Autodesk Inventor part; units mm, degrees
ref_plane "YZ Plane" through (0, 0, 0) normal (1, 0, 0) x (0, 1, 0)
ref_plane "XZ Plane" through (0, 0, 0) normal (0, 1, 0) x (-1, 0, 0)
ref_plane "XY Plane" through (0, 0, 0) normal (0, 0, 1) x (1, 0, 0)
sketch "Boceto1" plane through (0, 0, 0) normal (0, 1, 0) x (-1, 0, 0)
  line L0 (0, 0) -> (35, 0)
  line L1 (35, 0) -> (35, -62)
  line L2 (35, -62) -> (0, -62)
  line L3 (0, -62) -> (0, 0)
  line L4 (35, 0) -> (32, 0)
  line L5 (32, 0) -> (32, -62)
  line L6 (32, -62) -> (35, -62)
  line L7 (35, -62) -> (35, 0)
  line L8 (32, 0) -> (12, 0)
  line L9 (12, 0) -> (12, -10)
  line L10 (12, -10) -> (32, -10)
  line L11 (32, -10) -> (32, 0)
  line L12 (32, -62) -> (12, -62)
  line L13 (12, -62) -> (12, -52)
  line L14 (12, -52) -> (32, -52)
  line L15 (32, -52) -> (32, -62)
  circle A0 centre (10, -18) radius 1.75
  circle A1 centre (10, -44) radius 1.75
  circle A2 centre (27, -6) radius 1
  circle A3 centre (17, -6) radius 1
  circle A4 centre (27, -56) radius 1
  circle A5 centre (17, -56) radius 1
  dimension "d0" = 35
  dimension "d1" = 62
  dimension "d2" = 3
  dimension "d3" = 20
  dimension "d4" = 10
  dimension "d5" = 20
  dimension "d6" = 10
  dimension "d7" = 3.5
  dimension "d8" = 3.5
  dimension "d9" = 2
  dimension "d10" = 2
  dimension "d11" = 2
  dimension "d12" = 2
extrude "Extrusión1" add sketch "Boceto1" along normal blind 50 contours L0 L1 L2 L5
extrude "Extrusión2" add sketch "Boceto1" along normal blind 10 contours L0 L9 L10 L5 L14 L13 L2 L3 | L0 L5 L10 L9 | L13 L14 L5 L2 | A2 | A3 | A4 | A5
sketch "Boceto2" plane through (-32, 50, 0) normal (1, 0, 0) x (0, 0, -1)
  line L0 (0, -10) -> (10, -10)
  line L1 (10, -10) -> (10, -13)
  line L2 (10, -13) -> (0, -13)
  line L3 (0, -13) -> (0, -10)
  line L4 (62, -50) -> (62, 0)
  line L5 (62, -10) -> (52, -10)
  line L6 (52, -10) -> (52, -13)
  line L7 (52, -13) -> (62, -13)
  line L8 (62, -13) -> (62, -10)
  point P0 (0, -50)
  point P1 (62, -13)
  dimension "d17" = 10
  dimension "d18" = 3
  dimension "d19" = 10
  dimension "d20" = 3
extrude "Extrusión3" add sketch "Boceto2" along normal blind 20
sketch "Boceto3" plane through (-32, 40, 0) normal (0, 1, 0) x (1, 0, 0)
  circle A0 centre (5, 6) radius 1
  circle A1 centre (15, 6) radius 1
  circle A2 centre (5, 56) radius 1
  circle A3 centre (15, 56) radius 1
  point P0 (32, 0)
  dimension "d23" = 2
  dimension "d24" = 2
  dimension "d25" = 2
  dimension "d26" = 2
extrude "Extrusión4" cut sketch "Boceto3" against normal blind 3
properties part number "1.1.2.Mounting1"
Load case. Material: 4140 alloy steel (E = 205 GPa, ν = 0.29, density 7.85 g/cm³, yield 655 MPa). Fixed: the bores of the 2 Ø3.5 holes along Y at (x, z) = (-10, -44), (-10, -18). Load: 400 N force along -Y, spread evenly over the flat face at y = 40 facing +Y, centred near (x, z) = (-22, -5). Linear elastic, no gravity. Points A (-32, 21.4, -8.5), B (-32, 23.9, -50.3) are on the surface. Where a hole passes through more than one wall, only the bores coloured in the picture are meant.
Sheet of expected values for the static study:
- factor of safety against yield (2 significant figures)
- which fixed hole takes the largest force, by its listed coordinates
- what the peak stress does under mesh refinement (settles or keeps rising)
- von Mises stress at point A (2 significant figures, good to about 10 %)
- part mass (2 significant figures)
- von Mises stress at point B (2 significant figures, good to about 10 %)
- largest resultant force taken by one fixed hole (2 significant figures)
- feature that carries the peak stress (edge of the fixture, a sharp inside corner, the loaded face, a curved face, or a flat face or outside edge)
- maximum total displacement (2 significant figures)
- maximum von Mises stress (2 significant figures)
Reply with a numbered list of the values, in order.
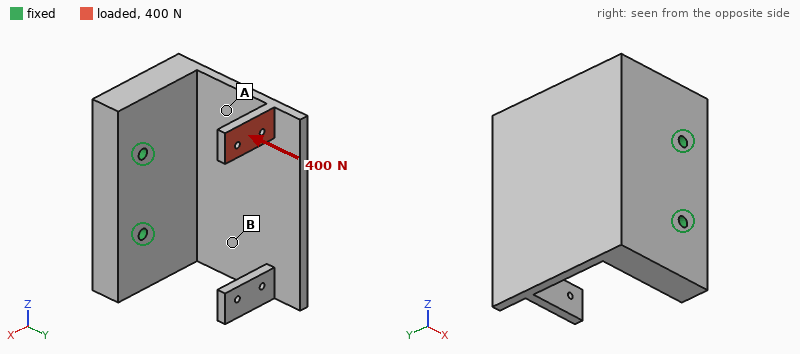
1. 1.9
2. (-10, -18)
3. settles
4. 73 MPa
5. 240 g
6. 30 MPa
7. 490 N
8. the loaded face
9. 0.31 mm
10. 350 MPa
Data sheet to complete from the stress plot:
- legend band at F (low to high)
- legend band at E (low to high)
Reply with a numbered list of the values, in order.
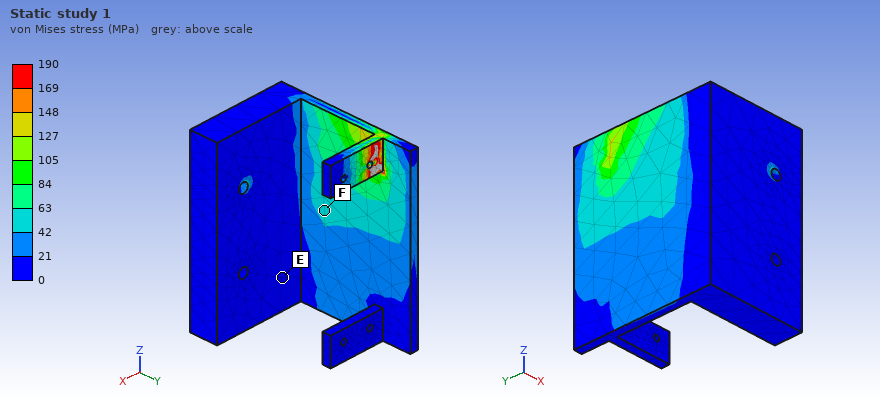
1. 42 to 63 MPa
2. 0 to 21 MPa
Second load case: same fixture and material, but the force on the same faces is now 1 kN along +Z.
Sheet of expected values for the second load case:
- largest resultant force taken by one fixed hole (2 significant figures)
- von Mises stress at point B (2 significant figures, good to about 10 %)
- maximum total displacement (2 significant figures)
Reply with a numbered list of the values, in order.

1. 1.2 kN
2. 20 MPa
3. 0.40 mm
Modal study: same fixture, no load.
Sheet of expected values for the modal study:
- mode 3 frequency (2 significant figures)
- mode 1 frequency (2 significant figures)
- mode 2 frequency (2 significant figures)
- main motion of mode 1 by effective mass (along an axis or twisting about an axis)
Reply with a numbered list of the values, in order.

1. 3800 Hz
2. 1200 Hz
3. 2000 Hz
4. along X
